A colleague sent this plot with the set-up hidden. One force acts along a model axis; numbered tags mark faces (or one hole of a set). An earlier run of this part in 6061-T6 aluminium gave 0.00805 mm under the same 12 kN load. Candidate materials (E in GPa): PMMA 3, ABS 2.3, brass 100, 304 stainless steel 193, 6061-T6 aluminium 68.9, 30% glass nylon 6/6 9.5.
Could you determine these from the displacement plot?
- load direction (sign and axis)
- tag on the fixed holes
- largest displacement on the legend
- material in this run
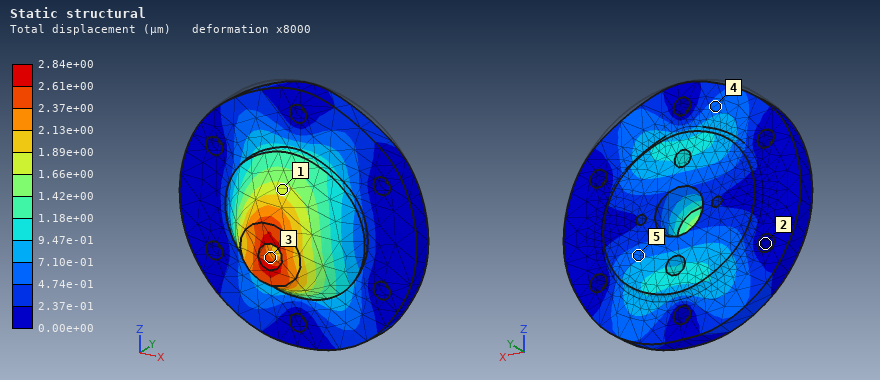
-Z
2
2.84e+00 µm
304 stainless steel
